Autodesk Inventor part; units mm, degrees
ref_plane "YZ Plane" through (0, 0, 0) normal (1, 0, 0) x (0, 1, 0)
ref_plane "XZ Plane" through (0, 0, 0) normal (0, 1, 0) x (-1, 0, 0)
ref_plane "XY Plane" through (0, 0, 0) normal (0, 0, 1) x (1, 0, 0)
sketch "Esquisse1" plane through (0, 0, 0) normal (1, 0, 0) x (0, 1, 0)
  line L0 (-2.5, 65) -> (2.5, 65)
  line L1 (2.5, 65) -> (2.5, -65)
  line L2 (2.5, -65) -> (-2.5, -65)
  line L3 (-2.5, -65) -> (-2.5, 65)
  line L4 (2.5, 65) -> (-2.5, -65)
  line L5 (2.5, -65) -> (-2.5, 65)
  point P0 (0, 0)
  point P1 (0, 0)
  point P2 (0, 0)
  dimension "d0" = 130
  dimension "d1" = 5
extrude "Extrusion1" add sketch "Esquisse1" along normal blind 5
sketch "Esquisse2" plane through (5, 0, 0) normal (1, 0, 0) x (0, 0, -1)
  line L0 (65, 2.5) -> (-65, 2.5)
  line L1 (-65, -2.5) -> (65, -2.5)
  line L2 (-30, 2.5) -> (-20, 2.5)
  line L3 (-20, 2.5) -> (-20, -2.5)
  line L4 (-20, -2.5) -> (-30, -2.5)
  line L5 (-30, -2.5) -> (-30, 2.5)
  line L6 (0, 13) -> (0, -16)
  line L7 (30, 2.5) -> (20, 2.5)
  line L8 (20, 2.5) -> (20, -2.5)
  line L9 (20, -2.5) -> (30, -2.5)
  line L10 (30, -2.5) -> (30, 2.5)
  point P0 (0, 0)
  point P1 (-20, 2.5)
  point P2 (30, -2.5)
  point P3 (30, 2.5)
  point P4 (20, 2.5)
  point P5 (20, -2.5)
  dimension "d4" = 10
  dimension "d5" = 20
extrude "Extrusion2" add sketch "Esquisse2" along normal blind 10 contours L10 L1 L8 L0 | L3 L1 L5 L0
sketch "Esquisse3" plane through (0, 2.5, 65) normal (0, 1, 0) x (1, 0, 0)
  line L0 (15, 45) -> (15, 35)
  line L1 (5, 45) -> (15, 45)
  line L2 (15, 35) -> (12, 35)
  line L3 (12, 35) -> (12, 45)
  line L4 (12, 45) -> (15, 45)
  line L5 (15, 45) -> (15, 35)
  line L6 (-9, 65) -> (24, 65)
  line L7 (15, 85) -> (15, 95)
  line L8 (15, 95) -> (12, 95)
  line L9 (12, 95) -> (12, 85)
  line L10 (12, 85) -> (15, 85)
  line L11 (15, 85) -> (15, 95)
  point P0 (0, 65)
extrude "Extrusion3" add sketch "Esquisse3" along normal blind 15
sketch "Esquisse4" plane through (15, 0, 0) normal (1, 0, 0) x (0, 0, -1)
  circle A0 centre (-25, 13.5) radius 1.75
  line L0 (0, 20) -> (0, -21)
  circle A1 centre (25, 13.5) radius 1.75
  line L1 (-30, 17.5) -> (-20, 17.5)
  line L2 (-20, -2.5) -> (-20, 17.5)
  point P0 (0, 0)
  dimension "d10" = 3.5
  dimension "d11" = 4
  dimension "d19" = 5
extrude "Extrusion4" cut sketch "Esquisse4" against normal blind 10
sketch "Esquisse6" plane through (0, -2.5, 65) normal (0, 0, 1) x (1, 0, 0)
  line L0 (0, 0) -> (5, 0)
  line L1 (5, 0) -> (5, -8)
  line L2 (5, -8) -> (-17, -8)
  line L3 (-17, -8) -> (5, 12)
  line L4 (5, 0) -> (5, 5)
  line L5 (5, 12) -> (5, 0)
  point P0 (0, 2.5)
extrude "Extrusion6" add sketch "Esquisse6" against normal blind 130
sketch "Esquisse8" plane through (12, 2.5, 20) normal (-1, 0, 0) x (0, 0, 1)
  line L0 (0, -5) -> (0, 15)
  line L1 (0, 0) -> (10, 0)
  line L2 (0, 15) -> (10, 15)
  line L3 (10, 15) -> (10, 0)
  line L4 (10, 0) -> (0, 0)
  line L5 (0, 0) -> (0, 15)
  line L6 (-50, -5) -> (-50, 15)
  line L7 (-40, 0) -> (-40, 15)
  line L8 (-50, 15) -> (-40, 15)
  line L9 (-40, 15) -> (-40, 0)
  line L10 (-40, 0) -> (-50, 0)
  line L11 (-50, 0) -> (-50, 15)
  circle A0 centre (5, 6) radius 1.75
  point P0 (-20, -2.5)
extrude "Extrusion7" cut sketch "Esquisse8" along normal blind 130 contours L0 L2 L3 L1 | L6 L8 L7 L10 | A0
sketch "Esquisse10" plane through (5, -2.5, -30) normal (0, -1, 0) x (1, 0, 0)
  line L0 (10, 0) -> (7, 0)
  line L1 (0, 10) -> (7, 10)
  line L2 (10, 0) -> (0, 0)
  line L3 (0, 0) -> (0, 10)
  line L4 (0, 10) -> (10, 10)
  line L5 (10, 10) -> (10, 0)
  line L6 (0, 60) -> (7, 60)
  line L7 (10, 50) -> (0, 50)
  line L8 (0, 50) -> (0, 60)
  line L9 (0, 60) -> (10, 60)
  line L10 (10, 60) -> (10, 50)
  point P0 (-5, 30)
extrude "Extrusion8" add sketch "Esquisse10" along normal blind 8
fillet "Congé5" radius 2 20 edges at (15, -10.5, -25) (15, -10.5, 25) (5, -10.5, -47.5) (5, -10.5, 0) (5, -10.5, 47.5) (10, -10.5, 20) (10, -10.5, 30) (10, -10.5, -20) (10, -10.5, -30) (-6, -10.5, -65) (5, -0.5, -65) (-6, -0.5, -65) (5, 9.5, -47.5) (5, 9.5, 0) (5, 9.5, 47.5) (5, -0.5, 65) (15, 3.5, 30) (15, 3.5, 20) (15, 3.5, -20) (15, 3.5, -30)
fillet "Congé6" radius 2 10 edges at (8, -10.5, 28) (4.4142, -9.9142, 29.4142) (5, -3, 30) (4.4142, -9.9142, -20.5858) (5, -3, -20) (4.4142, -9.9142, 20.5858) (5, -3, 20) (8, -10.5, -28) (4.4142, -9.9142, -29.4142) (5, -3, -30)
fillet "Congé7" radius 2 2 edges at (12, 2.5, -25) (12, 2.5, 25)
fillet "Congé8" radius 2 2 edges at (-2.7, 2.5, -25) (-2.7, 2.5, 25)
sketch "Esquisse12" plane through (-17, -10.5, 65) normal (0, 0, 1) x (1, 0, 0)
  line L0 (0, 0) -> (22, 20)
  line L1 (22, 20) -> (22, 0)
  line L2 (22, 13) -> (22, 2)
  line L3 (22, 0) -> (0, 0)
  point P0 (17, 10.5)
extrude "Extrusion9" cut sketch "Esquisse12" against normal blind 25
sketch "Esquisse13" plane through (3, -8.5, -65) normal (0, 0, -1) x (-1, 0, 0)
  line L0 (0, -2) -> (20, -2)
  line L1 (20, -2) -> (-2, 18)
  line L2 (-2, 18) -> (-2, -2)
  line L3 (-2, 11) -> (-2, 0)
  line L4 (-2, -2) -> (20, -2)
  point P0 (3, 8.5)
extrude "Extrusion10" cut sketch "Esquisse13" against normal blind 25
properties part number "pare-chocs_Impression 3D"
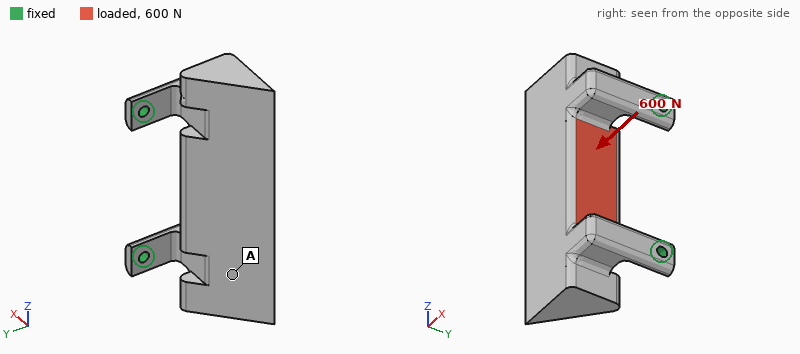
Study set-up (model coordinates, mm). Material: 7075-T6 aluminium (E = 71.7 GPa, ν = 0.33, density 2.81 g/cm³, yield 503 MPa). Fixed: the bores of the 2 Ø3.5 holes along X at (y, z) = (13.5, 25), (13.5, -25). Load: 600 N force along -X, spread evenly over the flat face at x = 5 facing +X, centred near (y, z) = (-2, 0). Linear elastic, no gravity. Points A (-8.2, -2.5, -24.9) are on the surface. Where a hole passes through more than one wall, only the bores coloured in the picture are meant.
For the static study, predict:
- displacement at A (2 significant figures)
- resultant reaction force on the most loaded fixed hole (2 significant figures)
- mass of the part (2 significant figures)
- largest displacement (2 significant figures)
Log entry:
0.46 mm
300 N
56 g
0.68 mm
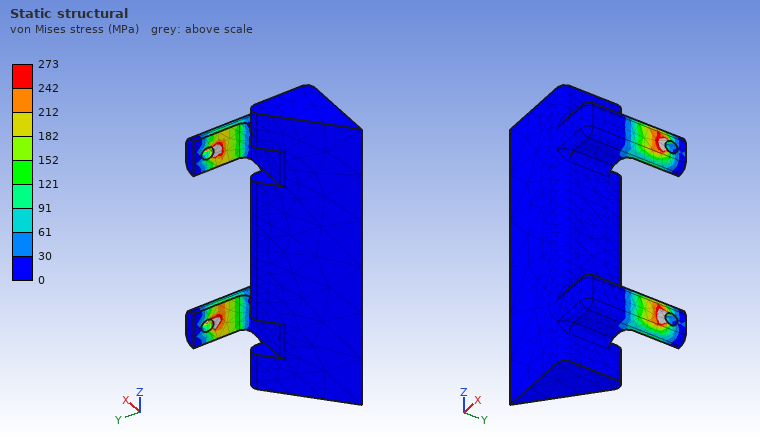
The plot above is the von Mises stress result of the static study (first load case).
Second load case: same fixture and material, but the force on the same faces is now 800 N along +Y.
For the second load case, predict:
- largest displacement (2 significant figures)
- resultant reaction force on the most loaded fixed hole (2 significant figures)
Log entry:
0.84 mm
400 N
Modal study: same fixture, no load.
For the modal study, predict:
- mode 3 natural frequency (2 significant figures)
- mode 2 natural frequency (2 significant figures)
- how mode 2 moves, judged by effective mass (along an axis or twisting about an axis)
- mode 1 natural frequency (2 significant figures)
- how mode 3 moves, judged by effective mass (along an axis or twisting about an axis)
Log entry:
3700 Hz
2500 Hz
along Z
570 Hz
along Z
